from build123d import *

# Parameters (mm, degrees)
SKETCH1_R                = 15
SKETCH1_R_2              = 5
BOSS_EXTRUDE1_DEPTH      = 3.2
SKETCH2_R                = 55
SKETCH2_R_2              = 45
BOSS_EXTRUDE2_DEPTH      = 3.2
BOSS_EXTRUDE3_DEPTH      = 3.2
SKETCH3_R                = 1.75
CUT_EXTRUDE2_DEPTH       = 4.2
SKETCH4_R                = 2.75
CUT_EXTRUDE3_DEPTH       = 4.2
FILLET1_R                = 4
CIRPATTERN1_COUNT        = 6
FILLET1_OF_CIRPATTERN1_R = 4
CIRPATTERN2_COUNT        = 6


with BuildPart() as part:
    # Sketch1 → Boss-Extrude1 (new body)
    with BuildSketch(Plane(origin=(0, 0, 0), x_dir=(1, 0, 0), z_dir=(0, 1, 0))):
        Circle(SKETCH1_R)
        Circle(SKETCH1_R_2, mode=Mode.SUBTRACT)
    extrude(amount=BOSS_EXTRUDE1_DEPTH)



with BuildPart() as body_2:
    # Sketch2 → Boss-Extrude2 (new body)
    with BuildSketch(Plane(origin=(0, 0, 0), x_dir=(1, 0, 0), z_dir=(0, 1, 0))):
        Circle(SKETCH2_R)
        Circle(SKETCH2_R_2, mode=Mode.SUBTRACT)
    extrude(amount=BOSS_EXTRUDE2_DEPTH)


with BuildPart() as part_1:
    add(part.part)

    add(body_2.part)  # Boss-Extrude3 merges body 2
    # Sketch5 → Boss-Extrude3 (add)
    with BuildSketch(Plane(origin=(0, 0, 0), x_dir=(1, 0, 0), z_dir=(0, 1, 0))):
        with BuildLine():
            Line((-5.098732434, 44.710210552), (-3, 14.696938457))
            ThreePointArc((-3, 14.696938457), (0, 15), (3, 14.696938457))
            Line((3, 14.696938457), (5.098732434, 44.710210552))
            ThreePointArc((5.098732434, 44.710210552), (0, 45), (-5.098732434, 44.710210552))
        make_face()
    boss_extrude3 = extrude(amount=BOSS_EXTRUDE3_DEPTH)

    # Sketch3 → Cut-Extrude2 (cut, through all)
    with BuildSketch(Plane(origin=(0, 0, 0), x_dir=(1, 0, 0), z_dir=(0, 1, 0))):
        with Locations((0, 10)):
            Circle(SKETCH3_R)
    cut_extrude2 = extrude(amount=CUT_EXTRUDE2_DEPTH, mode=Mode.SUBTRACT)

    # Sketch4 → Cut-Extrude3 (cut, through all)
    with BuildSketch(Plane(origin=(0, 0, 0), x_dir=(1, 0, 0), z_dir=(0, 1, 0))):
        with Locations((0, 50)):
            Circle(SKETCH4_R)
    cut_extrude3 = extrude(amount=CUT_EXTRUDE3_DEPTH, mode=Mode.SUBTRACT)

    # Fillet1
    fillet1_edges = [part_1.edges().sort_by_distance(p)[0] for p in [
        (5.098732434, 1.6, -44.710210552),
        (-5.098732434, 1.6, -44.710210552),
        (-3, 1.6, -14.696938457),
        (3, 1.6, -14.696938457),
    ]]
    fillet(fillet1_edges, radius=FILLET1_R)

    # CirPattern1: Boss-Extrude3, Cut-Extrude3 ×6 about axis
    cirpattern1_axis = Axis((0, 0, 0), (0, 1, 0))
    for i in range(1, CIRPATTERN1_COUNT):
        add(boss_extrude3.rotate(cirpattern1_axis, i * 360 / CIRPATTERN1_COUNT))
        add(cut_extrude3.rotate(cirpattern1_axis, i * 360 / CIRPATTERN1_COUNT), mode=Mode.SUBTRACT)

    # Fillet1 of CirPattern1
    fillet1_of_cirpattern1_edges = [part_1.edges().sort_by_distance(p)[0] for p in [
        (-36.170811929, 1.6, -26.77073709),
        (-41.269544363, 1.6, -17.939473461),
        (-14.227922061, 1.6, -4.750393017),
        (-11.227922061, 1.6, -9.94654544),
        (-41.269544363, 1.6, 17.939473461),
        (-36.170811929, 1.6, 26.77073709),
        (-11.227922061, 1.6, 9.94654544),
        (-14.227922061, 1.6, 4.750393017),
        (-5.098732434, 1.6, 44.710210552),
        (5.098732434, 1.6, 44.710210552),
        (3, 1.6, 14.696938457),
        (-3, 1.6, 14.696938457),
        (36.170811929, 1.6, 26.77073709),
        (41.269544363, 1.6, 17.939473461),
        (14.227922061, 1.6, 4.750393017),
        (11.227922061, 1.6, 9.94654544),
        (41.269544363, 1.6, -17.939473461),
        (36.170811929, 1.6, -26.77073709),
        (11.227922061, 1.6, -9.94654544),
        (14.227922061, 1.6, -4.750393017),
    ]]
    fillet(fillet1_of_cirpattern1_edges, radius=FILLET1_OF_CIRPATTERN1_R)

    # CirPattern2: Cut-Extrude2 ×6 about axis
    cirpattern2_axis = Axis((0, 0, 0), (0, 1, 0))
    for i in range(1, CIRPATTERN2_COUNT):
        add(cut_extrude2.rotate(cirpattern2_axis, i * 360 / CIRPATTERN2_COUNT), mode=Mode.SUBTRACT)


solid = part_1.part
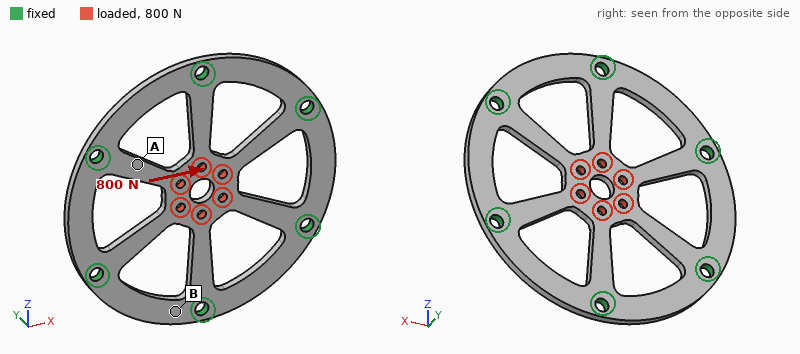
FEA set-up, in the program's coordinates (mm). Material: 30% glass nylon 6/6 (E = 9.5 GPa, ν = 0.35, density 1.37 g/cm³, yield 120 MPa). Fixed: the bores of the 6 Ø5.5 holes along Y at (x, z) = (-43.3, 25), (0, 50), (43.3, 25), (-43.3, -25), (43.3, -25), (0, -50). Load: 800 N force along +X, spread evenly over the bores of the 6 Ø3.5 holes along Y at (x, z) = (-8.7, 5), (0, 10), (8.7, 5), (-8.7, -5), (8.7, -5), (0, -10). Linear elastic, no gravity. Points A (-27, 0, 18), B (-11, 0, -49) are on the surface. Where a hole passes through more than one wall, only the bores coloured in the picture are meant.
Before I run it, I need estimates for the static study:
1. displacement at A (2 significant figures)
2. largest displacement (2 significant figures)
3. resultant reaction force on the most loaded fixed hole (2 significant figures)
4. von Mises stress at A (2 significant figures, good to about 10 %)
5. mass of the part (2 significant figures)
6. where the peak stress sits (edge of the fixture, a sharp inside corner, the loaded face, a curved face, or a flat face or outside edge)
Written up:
12 µm
40 µm
210 N
7.6 MPa
22 g
a sharp inside corner
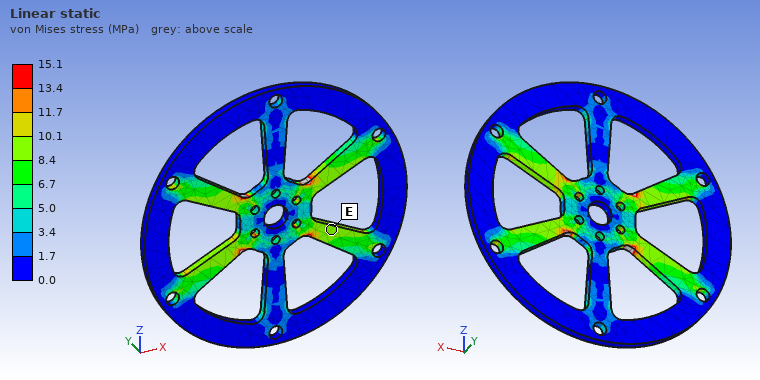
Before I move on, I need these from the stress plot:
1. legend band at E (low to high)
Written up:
8.4 to 10.1 MPa
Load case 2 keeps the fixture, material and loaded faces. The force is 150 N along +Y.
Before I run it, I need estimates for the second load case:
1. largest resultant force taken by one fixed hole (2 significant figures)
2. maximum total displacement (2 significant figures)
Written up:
25 N
0.70 mm
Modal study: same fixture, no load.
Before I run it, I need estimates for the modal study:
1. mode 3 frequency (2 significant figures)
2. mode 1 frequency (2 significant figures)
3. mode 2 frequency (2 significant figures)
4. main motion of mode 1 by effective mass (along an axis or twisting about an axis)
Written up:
2900 Hz
1200 Hz
2900 Hz
along Y
